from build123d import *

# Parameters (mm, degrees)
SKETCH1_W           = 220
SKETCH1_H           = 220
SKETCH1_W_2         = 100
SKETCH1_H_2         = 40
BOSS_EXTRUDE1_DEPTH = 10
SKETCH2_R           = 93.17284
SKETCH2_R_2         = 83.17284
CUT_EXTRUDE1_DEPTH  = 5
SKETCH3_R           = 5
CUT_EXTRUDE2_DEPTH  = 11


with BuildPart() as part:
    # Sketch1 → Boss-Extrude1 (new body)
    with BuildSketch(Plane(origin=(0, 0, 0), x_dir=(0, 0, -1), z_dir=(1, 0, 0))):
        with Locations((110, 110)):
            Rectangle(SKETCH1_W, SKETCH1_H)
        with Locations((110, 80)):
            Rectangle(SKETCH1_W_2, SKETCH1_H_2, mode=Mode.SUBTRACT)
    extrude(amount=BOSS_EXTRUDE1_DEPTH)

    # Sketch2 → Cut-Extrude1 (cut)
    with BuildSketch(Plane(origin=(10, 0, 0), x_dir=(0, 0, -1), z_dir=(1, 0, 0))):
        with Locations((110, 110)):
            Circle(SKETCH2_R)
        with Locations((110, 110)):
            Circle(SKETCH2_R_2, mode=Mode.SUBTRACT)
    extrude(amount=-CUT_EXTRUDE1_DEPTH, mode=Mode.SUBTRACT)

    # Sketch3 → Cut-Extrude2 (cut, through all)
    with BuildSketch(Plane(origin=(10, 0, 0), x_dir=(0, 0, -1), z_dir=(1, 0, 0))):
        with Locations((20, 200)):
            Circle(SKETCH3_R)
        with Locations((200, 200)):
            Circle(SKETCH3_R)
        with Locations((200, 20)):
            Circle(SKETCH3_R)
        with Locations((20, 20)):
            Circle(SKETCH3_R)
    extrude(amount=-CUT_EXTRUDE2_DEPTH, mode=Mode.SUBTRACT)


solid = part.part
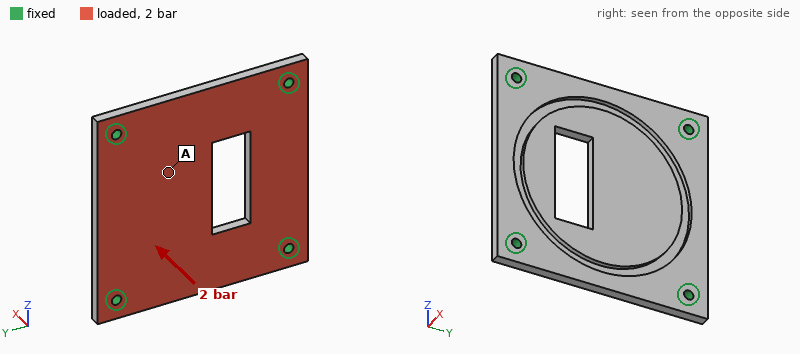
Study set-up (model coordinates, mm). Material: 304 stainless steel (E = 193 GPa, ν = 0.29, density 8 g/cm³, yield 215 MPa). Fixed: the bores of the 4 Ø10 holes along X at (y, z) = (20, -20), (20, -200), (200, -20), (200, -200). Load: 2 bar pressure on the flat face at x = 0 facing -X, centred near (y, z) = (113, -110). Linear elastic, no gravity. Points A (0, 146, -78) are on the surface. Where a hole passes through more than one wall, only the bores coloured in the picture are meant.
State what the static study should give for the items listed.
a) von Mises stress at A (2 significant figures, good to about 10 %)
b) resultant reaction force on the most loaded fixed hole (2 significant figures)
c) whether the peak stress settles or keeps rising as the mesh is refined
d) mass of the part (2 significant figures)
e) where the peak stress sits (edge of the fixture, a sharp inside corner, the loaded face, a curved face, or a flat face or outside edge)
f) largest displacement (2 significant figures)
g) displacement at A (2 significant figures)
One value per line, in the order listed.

13 MPa
2.3 kN
keeps rising
3.3 kg
edge of the fixture
0.12 mm
0.080 mm
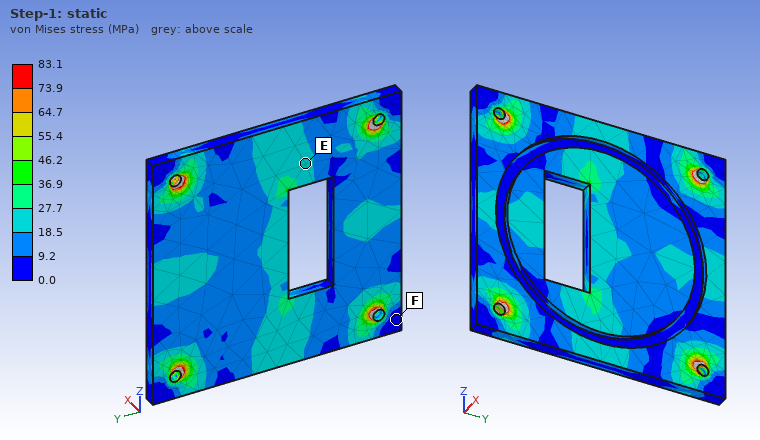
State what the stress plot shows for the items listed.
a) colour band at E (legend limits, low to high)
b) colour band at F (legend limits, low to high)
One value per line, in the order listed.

18.5 to 27.7 MPa
0.0 to 9.2 MPa
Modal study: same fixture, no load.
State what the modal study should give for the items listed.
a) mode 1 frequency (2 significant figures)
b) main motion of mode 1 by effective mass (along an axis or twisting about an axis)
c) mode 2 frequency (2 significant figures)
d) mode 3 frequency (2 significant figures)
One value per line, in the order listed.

1000 Hz
along X
1600 Hz
1600 Hz
